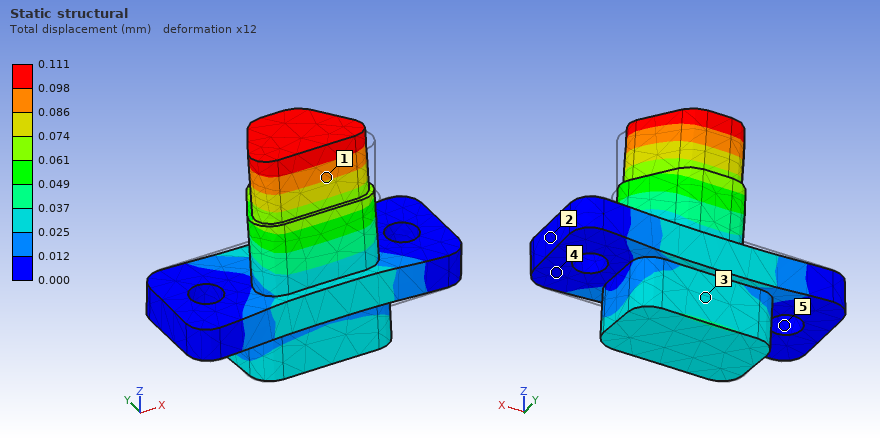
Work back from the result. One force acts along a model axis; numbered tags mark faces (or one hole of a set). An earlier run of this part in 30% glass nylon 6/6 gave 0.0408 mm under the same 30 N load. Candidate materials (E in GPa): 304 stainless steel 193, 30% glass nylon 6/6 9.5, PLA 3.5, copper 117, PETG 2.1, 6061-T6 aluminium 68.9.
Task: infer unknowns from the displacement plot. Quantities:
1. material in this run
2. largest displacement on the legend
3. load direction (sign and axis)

PLA
0.111 mm
+Y
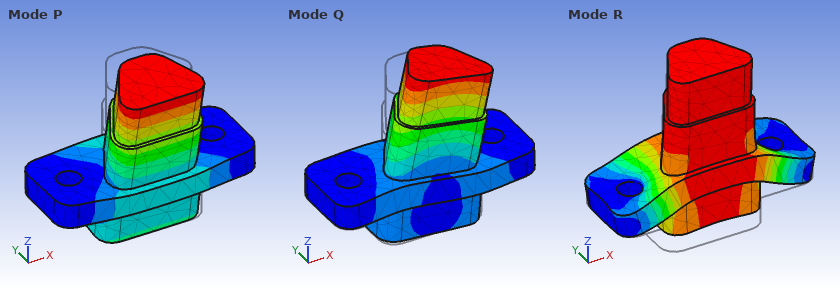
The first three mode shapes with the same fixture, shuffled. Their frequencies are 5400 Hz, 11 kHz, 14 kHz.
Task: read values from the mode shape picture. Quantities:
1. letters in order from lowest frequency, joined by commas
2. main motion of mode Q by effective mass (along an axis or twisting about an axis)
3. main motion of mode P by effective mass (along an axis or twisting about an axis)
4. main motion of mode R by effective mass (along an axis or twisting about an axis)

P, Q, R
along X
along Y
along Z
